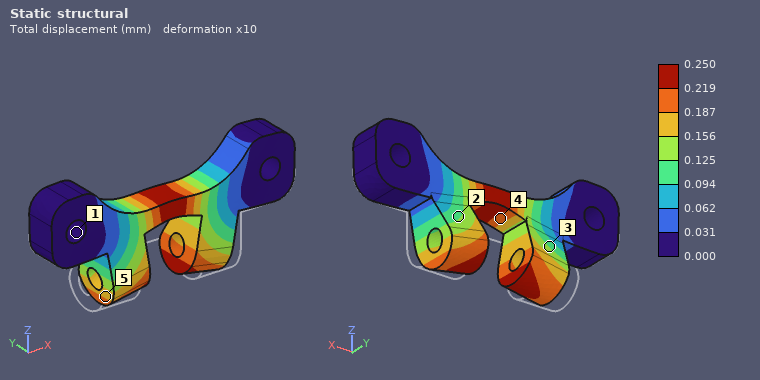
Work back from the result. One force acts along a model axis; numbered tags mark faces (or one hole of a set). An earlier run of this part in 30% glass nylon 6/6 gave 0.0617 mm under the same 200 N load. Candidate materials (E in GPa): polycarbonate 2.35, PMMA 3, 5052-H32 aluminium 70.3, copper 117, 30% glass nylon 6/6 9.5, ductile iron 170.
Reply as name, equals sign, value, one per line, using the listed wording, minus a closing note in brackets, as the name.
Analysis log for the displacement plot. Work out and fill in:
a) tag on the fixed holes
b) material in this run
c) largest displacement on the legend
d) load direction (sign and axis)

tag on the fixed holes = 1
material in this run = polycarbonate
largest displacement on the legend = 0.250 mm
load direction = +Z
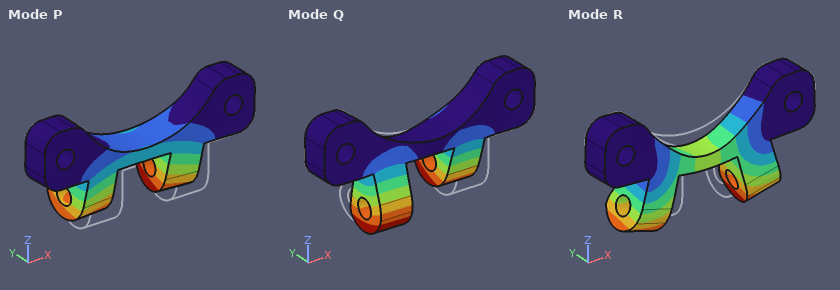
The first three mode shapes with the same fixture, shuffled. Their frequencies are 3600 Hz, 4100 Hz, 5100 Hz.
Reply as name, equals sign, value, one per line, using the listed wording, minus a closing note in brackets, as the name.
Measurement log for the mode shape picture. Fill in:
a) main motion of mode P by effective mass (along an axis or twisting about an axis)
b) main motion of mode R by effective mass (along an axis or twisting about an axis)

main motion of mode P by effective mass = along Y
main motion of mode R by effective mass = along Z
